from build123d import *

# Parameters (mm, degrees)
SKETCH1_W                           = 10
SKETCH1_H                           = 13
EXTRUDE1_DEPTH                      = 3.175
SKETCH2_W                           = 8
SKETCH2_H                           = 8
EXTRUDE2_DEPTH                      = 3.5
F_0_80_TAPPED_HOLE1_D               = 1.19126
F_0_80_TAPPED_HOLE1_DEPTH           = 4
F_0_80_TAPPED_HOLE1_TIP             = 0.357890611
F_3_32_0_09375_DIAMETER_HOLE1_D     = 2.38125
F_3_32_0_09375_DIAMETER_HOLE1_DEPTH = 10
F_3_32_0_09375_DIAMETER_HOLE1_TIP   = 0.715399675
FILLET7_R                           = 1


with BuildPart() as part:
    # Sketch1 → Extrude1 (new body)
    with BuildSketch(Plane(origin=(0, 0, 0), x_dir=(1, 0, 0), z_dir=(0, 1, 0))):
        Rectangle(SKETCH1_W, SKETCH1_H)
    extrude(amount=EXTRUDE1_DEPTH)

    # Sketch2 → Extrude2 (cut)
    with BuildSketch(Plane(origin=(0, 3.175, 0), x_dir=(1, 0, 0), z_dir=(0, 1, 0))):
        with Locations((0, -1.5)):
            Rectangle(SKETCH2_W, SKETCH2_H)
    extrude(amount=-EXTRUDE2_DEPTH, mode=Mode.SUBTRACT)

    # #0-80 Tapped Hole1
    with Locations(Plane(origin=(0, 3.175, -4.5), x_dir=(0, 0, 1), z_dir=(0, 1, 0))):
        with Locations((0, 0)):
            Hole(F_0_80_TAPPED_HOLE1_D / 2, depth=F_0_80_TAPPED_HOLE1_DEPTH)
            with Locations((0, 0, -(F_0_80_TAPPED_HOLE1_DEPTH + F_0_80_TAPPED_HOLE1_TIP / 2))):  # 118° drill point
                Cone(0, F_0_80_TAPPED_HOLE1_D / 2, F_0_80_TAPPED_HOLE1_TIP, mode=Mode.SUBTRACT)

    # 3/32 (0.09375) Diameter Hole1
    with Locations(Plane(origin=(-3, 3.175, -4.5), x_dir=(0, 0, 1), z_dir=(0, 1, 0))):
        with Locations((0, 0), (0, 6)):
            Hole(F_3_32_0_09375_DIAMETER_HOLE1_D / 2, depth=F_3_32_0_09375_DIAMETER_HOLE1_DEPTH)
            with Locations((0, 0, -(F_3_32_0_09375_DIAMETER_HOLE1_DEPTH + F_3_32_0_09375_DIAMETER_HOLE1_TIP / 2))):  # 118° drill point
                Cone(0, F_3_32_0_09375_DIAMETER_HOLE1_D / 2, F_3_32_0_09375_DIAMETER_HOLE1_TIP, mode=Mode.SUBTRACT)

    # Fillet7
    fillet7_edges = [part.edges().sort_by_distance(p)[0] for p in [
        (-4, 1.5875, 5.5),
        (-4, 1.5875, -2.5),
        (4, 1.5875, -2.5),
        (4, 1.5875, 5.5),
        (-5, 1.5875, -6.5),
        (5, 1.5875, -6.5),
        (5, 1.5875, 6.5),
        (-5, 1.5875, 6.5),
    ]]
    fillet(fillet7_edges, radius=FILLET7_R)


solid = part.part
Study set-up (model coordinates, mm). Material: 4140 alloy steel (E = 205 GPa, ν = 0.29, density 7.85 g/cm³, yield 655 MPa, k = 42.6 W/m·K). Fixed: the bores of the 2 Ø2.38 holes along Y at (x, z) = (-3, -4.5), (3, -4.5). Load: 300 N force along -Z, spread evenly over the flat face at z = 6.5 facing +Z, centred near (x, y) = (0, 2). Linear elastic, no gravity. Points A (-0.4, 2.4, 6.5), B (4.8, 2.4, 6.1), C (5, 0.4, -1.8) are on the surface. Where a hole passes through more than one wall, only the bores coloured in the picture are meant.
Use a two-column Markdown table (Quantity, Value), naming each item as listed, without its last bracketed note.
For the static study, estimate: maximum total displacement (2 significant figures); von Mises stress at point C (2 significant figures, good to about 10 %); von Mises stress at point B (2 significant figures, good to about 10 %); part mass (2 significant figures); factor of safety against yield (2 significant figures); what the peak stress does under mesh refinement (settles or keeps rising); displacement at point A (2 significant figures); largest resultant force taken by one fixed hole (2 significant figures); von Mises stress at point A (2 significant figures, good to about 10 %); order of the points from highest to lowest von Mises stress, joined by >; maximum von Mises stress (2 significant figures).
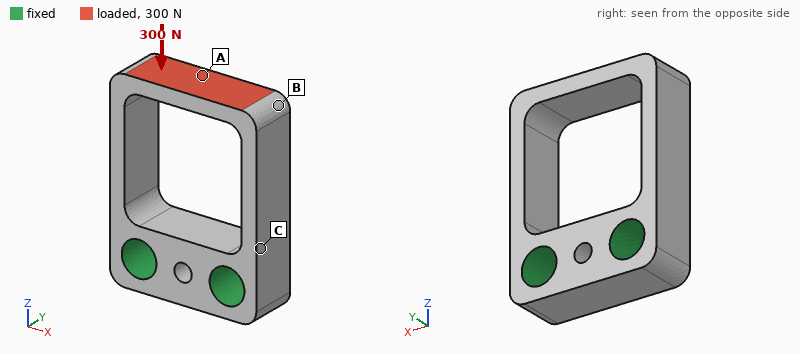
| Quantity | Value |
|---|---|
| maximum total displacement | 25 µm |
| von Mises stress at point C | 150 MPa |
| von Mises stress at point B | 56 MPa |
| part mass | 1.4 g |
| factor of safety against yield | 1.7 |
| what the peak stress does under mesh refinement | settles |
| displacement at point A | 24 µm |
| largest resultant force taken by one fixed hole | 150 N |
| von Mises stress at point A | 330 MPa |
| order of the points from highest to lowest von Mises stress, joined by > | A > C > B |
| maximum von Mises stress | 370 MPa |
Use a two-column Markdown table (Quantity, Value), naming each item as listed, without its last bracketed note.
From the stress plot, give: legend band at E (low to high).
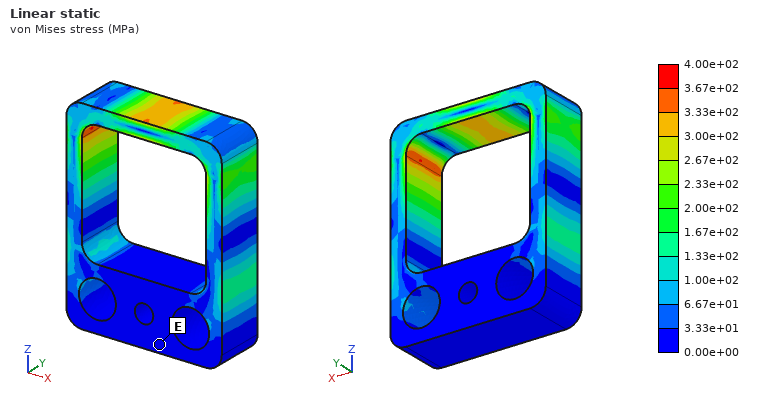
| Quantity | Value |
|---|---|
| legend band at E | 0.00e+00 to 3.33e+01 MPa |
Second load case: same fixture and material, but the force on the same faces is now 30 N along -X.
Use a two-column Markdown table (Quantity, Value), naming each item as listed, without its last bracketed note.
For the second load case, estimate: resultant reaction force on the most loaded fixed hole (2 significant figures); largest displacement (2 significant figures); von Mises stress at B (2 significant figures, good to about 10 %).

| Quantity | Value |
|---|---|
| resultant reaction force on the most loaded fixed hole | 24 N |
| largest displacement | 17 µm |
| von Mises stress at B | 23 MPa |
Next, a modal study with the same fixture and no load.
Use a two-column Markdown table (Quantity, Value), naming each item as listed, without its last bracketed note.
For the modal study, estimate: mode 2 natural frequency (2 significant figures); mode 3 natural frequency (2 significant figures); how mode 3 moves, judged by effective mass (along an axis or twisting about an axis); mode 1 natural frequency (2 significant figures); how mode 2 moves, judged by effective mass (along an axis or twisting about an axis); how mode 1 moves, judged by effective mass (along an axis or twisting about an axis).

| Quantity | Value |
|---|---|
| mode 2 natural frequency | 16 kHz |
| mode 3 natural frequency | 26 kHz |
| how mode 3 moves, judged by effective mass | twisting about Z |
| mode 1 natural frequency | 11 kHz |
| how mode 2 moves, judged by effective mass | along Y |
| how mode 1 moves, judged by effective mass | along X |
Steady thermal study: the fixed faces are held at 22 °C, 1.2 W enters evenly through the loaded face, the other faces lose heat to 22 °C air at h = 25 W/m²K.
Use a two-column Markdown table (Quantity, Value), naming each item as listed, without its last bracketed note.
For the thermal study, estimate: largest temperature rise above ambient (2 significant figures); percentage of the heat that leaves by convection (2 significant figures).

| Quantity | Value |
|---|---|
| largest temperature rise above ambient | 44 K |
| percentage of the heat that leaves by convection | 9.6 % |
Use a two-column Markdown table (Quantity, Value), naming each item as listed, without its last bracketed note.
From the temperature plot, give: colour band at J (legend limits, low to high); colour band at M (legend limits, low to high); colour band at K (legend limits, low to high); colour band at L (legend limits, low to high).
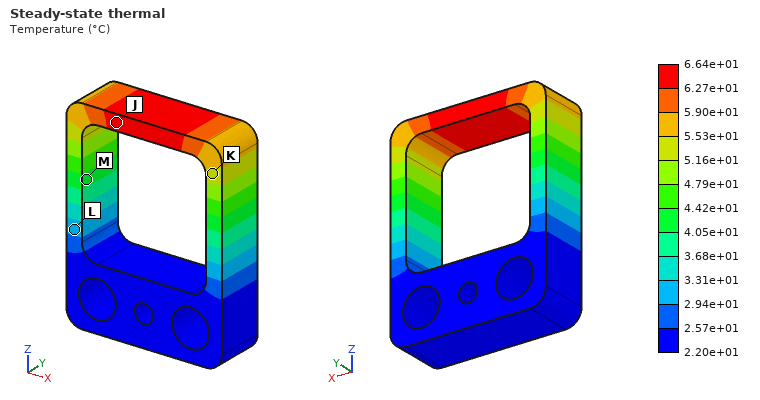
| Quantity | Value |
|---|---|
| colour band at J | 6.27e+01 to 6.64e+01 °C |
| colour band at M | 4.05e+01 to 4.42e+01 °C |
| colour band at K | 5.16e+01 to 5.53e+01 °C |
| colour band at L | 2.94e+01 to 3.31e+01 °C |
